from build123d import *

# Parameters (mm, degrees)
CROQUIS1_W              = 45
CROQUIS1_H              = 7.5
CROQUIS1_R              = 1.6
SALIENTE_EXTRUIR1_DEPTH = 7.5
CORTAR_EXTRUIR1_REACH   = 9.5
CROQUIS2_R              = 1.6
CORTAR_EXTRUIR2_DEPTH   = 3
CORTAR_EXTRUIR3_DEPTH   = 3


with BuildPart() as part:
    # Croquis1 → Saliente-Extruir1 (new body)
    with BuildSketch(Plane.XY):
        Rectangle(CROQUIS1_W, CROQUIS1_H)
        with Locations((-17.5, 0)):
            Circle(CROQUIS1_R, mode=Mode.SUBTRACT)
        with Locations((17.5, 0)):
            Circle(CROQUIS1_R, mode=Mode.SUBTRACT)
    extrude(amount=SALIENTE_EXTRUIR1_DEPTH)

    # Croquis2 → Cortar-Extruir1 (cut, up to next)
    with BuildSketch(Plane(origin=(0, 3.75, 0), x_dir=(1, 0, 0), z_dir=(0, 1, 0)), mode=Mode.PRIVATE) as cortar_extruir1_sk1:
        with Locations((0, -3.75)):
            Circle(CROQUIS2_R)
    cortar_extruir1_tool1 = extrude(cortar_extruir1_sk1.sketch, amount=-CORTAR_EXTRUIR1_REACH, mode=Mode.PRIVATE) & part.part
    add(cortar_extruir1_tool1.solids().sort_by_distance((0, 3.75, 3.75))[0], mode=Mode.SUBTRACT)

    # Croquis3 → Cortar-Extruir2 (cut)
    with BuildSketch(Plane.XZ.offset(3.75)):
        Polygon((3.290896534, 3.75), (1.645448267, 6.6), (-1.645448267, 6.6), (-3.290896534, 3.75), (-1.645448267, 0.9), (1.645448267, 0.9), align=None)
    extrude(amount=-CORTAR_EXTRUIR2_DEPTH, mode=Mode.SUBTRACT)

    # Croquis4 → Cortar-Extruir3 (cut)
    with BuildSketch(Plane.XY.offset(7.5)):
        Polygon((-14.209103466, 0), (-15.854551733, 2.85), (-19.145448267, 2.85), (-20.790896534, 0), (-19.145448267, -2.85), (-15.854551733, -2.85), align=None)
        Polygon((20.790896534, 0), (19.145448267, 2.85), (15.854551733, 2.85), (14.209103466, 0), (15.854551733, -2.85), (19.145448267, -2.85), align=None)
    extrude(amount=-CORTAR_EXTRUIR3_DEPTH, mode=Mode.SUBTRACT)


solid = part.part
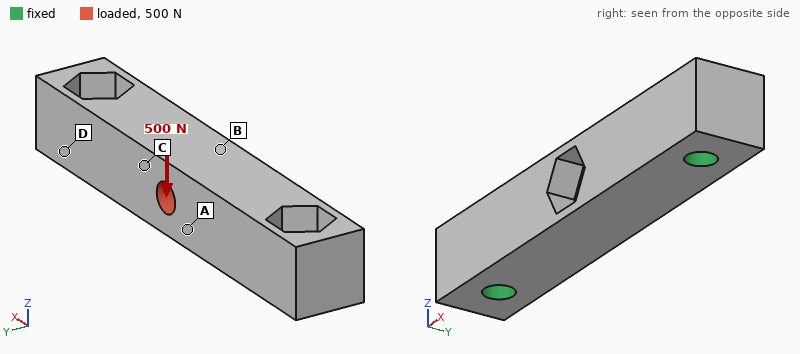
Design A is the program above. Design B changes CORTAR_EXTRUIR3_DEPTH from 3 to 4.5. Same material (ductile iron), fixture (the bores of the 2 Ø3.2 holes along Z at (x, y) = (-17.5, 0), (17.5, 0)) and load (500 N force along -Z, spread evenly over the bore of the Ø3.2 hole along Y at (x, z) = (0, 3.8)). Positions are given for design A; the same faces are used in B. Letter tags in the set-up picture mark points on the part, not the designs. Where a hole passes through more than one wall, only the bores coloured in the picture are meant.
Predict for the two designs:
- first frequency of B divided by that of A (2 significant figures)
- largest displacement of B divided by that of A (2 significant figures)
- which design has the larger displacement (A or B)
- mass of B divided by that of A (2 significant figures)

0.86
1.2
B
0.97
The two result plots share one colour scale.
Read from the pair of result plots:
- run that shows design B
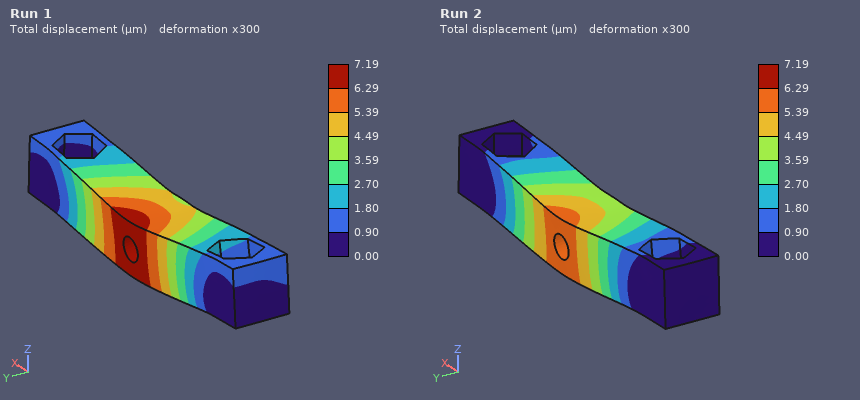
Run 1
